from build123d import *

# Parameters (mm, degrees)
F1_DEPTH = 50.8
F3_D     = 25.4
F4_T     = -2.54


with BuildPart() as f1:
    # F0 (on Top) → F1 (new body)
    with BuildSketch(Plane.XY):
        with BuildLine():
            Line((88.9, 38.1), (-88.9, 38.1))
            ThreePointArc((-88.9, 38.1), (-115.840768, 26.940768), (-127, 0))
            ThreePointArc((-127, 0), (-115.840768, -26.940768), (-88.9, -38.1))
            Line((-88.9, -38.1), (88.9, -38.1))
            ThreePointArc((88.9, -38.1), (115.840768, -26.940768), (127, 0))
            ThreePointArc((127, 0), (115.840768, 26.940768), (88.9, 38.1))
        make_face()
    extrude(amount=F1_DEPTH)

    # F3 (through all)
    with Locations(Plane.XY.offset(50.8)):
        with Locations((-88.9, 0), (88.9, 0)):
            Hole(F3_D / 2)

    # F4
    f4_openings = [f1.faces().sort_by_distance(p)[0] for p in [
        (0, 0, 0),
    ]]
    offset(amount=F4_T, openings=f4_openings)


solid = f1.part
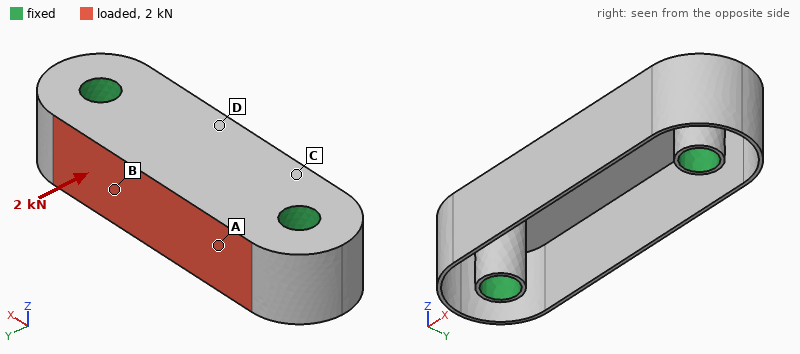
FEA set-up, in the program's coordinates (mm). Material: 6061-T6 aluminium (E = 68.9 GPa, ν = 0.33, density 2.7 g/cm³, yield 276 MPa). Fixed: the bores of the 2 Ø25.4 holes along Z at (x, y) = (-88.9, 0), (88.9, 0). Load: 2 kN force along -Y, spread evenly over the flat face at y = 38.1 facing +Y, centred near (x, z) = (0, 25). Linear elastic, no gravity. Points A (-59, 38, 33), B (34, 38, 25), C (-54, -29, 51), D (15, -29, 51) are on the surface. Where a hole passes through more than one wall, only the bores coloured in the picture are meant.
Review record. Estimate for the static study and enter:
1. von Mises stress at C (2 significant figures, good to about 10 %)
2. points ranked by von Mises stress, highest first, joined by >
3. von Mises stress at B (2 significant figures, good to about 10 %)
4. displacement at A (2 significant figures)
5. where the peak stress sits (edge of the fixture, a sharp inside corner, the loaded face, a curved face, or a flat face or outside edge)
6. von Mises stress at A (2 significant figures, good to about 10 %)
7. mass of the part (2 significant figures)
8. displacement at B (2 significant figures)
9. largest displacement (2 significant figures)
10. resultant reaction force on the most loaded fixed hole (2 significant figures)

34 MPa
A > B > C > D
55 MPa
0.78 mm
a flat face or outside edge
83 MPa
370 g
1.4 mm
3.2 mm
1.0 kN
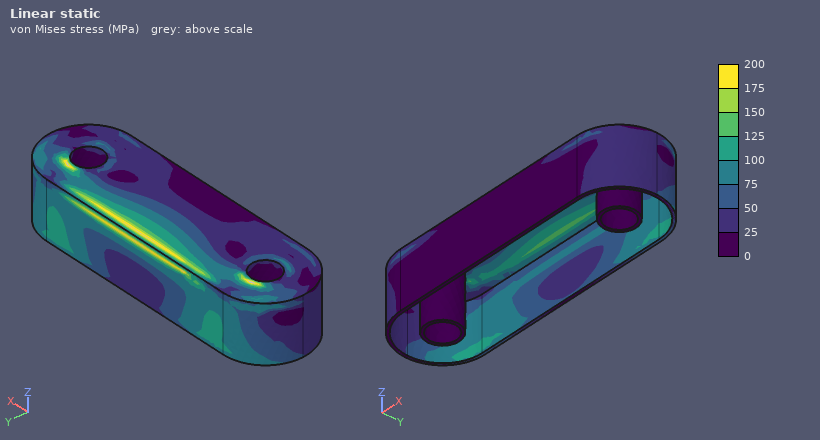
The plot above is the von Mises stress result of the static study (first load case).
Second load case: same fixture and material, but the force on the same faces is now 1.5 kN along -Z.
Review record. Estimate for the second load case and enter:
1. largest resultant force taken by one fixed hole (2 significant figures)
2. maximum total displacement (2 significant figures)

890 N
0.81 mm
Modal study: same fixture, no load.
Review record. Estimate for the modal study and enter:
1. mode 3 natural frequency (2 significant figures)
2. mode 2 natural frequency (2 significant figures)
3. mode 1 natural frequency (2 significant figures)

770 Hz
630 Hz
620 Hz
